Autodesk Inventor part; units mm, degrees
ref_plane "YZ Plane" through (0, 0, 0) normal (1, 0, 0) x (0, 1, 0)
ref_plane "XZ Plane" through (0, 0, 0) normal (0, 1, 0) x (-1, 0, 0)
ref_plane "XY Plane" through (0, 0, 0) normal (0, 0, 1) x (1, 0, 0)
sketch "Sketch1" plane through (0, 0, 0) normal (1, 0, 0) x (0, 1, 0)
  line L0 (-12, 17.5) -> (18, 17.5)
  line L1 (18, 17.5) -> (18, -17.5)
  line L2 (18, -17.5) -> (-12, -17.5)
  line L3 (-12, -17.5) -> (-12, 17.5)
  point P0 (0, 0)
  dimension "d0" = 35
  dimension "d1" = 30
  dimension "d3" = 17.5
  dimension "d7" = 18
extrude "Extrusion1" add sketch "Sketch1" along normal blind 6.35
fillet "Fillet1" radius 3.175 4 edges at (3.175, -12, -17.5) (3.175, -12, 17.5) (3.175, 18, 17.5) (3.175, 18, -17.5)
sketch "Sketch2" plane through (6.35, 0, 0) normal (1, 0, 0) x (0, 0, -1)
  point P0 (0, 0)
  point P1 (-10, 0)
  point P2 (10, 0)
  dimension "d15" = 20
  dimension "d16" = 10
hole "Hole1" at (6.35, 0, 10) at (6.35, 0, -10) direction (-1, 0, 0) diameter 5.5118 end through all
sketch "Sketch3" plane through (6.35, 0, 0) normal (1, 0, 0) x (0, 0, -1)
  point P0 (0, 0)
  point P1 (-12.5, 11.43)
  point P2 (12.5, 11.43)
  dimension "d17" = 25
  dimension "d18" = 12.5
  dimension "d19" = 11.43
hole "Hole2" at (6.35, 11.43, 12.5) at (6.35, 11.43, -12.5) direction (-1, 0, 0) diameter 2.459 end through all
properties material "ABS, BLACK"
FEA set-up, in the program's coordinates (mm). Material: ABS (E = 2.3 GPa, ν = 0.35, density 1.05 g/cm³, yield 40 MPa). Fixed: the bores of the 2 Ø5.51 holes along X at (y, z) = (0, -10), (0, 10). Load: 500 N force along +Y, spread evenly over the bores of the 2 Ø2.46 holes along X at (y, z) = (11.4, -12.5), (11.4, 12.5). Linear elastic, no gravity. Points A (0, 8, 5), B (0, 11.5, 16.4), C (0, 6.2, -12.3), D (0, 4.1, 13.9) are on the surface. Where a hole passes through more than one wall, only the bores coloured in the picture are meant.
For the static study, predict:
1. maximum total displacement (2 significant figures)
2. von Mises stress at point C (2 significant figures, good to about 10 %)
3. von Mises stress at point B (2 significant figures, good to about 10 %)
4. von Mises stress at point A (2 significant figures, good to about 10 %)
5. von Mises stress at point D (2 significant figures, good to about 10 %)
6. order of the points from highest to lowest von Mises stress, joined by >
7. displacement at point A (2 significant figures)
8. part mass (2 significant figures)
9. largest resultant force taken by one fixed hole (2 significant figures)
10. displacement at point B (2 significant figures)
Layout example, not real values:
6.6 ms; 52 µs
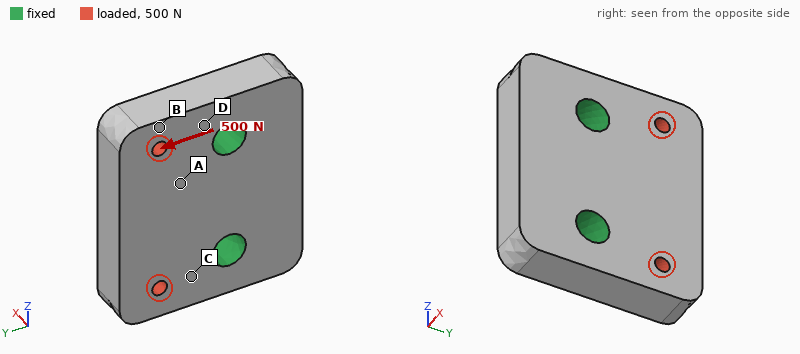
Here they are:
24 µm; 4.5 MPa; 1.7 MPa; 0.89 MPa; 3.1 MPa; C > D > B > A; 4.7 µm; 6.6 g; 250 N; 17 µm
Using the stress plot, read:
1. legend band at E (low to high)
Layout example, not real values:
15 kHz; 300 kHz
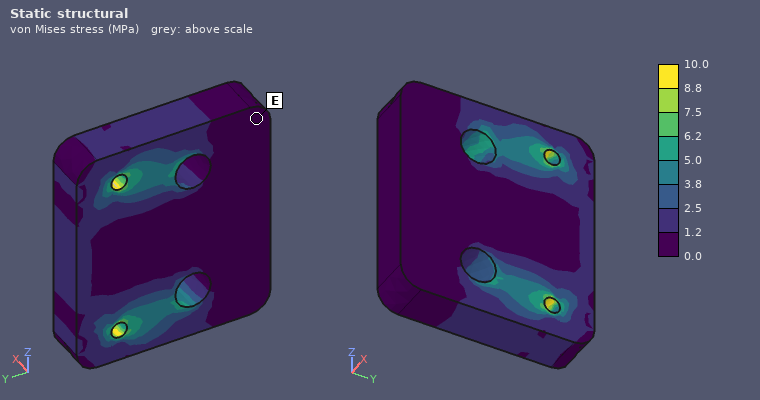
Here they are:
0.0 to 1.2 MPa
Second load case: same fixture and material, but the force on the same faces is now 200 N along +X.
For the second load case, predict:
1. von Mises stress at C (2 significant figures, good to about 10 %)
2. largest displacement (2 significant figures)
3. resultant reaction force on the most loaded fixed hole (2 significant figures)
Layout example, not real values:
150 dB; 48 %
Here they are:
5.1 MPa; 0.11 mm; 100 N
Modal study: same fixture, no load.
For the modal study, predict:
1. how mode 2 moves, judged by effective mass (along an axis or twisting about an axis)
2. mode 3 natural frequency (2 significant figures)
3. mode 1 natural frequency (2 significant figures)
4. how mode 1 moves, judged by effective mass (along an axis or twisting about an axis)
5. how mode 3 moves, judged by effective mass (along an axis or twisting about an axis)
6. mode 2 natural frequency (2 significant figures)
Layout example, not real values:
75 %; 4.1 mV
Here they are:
twisting about Y; 10 kHz; 4800 Hz; along X; along X; 6900 Hz
